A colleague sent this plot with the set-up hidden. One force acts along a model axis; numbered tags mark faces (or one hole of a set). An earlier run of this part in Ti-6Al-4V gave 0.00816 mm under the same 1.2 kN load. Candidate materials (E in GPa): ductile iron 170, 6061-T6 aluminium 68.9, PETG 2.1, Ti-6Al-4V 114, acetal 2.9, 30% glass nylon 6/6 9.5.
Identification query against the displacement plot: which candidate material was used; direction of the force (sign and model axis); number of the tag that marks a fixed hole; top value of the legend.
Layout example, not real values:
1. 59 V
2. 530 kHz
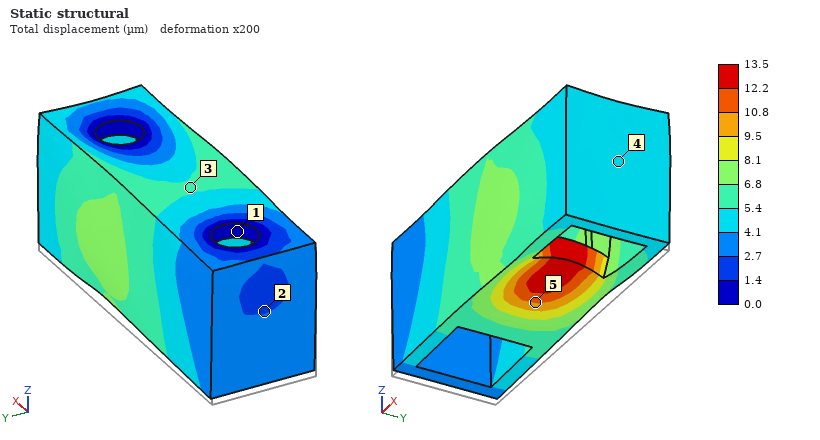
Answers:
1. 6061-T6 aluminium
2. +Z
3. 1
4. 13.5 µm
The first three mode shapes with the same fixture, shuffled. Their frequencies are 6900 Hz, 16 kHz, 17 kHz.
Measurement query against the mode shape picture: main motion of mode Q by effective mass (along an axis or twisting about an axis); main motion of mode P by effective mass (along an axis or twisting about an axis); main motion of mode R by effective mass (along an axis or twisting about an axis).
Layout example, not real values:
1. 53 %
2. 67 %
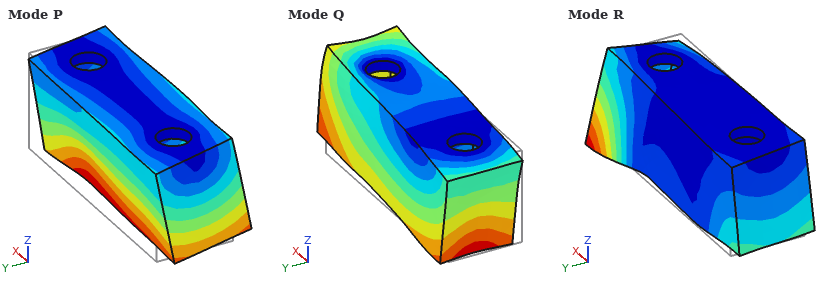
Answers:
1. along X
2. along Y
3. twisting about Z
